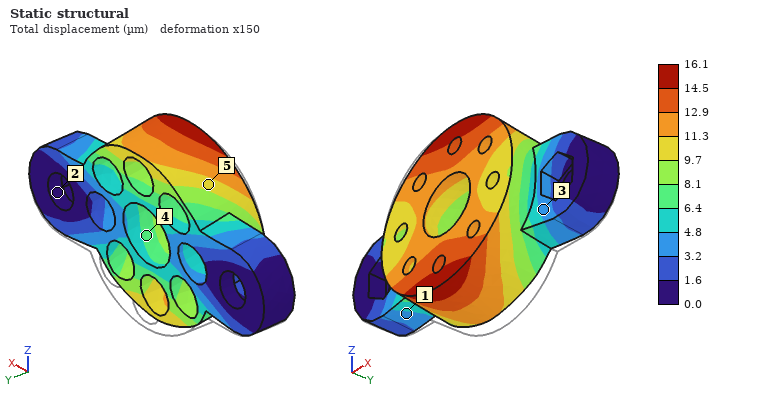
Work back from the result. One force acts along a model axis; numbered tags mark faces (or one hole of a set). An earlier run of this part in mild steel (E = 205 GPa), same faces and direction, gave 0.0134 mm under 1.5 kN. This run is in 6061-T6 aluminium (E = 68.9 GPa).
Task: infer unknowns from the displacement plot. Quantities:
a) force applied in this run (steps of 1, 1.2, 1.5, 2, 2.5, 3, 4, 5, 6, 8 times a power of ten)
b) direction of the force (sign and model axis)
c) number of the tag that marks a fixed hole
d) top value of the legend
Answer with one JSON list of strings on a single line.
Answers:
["600 N", "+Z", "2", "16.1 µm"]
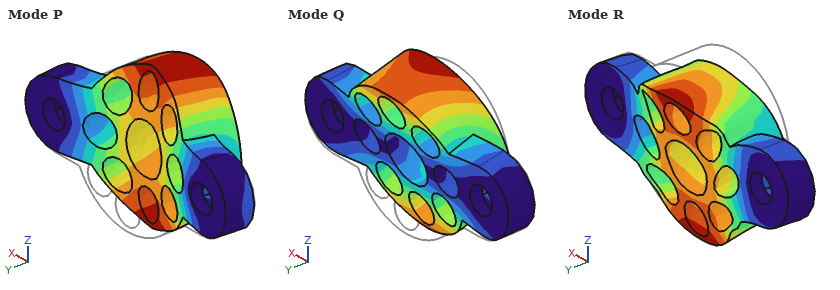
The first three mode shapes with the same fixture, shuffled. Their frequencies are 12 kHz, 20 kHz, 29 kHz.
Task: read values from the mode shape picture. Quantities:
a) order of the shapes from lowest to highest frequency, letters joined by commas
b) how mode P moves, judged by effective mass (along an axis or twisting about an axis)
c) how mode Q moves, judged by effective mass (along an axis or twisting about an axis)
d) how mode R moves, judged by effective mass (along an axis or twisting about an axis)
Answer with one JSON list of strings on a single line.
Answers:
["Q, P, R", "along Y", "along Z", "along Z"]
